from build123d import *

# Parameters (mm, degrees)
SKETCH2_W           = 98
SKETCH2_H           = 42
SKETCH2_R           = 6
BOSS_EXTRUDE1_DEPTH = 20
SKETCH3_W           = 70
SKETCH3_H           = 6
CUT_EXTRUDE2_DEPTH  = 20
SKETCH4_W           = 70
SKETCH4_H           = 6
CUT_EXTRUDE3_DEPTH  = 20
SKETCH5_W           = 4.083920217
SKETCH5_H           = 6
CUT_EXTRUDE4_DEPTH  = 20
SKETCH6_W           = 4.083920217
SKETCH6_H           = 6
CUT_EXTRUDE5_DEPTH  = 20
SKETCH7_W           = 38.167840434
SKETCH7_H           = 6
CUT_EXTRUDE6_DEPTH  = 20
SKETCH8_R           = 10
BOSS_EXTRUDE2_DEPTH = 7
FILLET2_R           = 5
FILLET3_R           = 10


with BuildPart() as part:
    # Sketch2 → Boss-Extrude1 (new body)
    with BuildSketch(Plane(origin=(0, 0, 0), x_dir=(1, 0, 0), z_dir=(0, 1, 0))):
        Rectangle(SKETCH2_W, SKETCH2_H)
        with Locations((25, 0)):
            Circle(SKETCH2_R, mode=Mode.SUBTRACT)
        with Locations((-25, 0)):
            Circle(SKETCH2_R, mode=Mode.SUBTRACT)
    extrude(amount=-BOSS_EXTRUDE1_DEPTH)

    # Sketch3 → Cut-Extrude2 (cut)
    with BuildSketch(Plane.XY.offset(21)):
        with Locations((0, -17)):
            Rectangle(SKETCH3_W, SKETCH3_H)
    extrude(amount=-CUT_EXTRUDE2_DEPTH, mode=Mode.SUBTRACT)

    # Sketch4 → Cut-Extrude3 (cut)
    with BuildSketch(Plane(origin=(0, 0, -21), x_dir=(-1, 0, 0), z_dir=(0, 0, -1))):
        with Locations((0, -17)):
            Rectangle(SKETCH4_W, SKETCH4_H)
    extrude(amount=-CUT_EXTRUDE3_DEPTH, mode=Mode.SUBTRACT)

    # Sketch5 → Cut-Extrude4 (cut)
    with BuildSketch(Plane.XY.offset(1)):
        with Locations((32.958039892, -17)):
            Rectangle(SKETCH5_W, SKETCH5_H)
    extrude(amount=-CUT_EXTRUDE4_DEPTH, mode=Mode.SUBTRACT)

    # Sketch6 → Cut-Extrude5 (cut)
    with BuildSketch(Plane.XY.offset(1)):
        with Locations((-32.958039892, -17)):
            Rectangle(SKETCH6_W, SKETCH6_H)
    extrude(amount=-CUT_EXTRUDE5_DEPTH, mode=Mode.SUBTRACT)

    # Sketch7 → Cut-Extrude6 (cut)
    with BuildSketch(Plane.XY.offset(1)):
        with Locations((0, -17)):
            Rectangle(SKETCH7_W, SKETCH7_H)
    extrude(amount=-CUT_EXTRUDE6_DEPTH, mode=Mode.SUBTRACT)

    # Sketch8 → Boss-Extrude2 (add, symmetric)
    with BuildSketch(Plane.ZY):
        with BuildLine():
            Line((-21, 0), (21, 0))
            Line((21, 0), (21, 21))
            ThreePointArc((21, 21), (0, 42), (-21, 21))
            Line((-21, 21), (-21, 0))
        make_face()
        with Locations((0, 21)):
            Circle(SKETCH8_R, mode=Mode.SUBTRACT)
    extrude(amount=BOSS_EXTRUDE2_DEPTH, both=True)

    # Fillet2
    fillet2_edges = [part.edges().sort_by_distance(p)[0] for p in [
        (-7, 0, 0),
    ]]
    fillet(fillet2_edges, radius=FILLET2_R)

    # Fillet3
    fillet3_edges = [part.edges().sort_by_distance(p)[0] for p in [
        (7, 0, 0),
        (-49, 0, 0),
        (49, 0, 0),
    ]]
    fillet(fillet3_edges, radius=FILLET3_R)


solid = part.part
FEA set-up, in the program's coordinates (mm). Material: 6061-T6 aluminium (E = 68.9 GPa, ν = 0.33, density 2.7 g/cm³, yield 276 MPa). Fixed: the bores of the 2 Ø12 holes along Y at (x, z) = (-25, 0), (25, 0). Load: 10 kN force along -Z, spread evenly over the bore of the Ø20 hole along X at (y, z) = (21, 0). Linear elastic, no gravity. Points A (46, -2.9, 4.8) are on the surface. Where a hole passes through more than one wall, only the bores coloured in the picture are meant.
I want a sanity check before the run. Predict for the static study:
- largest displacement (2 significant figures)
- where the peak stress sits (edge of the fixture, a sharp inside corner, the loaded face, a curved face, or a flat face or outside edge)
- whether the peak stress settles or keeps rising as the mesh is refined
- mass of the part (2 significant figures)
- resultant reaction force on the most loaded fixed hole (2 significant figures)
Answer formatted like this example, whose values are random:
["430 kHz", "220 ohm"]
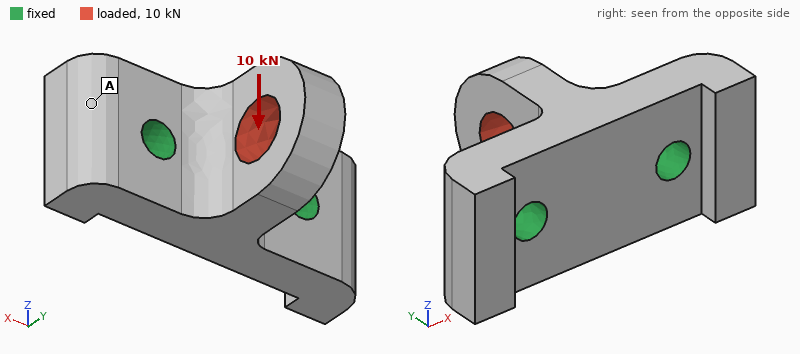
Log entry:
["0.17 mm", "edge of the fixture", "keeps rising", "210 g", "5.2 kN"]
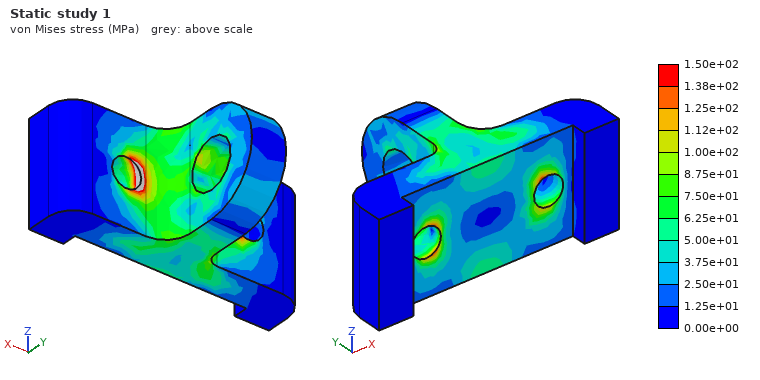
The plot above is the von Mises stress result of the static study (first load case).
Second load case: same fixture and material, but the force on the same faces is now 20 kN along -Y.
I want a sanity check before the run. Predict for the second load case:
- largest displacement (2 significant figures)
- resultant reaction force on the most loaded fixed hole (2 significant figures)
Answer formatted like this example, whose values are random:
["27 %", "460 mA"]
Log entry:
["58 µm", "11 kN"]
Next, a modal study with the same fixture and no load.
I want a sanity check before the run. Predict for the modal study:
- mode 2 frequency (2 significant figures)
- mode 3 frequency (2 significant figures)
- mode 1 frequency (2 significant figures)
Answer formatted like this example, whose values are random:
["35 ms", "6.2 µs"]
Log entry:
["6500 Hz", "13 kHz", "6300 Hz"]
